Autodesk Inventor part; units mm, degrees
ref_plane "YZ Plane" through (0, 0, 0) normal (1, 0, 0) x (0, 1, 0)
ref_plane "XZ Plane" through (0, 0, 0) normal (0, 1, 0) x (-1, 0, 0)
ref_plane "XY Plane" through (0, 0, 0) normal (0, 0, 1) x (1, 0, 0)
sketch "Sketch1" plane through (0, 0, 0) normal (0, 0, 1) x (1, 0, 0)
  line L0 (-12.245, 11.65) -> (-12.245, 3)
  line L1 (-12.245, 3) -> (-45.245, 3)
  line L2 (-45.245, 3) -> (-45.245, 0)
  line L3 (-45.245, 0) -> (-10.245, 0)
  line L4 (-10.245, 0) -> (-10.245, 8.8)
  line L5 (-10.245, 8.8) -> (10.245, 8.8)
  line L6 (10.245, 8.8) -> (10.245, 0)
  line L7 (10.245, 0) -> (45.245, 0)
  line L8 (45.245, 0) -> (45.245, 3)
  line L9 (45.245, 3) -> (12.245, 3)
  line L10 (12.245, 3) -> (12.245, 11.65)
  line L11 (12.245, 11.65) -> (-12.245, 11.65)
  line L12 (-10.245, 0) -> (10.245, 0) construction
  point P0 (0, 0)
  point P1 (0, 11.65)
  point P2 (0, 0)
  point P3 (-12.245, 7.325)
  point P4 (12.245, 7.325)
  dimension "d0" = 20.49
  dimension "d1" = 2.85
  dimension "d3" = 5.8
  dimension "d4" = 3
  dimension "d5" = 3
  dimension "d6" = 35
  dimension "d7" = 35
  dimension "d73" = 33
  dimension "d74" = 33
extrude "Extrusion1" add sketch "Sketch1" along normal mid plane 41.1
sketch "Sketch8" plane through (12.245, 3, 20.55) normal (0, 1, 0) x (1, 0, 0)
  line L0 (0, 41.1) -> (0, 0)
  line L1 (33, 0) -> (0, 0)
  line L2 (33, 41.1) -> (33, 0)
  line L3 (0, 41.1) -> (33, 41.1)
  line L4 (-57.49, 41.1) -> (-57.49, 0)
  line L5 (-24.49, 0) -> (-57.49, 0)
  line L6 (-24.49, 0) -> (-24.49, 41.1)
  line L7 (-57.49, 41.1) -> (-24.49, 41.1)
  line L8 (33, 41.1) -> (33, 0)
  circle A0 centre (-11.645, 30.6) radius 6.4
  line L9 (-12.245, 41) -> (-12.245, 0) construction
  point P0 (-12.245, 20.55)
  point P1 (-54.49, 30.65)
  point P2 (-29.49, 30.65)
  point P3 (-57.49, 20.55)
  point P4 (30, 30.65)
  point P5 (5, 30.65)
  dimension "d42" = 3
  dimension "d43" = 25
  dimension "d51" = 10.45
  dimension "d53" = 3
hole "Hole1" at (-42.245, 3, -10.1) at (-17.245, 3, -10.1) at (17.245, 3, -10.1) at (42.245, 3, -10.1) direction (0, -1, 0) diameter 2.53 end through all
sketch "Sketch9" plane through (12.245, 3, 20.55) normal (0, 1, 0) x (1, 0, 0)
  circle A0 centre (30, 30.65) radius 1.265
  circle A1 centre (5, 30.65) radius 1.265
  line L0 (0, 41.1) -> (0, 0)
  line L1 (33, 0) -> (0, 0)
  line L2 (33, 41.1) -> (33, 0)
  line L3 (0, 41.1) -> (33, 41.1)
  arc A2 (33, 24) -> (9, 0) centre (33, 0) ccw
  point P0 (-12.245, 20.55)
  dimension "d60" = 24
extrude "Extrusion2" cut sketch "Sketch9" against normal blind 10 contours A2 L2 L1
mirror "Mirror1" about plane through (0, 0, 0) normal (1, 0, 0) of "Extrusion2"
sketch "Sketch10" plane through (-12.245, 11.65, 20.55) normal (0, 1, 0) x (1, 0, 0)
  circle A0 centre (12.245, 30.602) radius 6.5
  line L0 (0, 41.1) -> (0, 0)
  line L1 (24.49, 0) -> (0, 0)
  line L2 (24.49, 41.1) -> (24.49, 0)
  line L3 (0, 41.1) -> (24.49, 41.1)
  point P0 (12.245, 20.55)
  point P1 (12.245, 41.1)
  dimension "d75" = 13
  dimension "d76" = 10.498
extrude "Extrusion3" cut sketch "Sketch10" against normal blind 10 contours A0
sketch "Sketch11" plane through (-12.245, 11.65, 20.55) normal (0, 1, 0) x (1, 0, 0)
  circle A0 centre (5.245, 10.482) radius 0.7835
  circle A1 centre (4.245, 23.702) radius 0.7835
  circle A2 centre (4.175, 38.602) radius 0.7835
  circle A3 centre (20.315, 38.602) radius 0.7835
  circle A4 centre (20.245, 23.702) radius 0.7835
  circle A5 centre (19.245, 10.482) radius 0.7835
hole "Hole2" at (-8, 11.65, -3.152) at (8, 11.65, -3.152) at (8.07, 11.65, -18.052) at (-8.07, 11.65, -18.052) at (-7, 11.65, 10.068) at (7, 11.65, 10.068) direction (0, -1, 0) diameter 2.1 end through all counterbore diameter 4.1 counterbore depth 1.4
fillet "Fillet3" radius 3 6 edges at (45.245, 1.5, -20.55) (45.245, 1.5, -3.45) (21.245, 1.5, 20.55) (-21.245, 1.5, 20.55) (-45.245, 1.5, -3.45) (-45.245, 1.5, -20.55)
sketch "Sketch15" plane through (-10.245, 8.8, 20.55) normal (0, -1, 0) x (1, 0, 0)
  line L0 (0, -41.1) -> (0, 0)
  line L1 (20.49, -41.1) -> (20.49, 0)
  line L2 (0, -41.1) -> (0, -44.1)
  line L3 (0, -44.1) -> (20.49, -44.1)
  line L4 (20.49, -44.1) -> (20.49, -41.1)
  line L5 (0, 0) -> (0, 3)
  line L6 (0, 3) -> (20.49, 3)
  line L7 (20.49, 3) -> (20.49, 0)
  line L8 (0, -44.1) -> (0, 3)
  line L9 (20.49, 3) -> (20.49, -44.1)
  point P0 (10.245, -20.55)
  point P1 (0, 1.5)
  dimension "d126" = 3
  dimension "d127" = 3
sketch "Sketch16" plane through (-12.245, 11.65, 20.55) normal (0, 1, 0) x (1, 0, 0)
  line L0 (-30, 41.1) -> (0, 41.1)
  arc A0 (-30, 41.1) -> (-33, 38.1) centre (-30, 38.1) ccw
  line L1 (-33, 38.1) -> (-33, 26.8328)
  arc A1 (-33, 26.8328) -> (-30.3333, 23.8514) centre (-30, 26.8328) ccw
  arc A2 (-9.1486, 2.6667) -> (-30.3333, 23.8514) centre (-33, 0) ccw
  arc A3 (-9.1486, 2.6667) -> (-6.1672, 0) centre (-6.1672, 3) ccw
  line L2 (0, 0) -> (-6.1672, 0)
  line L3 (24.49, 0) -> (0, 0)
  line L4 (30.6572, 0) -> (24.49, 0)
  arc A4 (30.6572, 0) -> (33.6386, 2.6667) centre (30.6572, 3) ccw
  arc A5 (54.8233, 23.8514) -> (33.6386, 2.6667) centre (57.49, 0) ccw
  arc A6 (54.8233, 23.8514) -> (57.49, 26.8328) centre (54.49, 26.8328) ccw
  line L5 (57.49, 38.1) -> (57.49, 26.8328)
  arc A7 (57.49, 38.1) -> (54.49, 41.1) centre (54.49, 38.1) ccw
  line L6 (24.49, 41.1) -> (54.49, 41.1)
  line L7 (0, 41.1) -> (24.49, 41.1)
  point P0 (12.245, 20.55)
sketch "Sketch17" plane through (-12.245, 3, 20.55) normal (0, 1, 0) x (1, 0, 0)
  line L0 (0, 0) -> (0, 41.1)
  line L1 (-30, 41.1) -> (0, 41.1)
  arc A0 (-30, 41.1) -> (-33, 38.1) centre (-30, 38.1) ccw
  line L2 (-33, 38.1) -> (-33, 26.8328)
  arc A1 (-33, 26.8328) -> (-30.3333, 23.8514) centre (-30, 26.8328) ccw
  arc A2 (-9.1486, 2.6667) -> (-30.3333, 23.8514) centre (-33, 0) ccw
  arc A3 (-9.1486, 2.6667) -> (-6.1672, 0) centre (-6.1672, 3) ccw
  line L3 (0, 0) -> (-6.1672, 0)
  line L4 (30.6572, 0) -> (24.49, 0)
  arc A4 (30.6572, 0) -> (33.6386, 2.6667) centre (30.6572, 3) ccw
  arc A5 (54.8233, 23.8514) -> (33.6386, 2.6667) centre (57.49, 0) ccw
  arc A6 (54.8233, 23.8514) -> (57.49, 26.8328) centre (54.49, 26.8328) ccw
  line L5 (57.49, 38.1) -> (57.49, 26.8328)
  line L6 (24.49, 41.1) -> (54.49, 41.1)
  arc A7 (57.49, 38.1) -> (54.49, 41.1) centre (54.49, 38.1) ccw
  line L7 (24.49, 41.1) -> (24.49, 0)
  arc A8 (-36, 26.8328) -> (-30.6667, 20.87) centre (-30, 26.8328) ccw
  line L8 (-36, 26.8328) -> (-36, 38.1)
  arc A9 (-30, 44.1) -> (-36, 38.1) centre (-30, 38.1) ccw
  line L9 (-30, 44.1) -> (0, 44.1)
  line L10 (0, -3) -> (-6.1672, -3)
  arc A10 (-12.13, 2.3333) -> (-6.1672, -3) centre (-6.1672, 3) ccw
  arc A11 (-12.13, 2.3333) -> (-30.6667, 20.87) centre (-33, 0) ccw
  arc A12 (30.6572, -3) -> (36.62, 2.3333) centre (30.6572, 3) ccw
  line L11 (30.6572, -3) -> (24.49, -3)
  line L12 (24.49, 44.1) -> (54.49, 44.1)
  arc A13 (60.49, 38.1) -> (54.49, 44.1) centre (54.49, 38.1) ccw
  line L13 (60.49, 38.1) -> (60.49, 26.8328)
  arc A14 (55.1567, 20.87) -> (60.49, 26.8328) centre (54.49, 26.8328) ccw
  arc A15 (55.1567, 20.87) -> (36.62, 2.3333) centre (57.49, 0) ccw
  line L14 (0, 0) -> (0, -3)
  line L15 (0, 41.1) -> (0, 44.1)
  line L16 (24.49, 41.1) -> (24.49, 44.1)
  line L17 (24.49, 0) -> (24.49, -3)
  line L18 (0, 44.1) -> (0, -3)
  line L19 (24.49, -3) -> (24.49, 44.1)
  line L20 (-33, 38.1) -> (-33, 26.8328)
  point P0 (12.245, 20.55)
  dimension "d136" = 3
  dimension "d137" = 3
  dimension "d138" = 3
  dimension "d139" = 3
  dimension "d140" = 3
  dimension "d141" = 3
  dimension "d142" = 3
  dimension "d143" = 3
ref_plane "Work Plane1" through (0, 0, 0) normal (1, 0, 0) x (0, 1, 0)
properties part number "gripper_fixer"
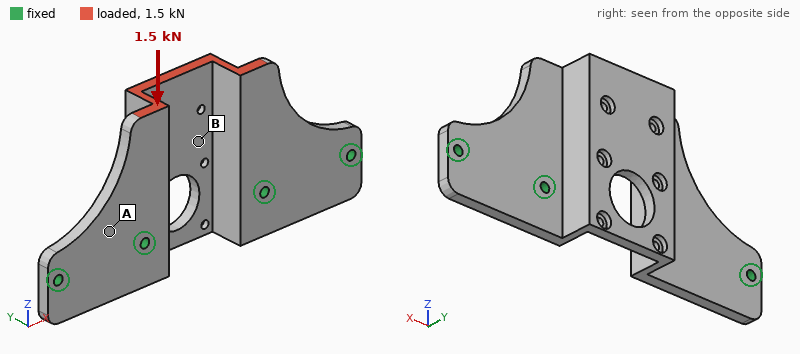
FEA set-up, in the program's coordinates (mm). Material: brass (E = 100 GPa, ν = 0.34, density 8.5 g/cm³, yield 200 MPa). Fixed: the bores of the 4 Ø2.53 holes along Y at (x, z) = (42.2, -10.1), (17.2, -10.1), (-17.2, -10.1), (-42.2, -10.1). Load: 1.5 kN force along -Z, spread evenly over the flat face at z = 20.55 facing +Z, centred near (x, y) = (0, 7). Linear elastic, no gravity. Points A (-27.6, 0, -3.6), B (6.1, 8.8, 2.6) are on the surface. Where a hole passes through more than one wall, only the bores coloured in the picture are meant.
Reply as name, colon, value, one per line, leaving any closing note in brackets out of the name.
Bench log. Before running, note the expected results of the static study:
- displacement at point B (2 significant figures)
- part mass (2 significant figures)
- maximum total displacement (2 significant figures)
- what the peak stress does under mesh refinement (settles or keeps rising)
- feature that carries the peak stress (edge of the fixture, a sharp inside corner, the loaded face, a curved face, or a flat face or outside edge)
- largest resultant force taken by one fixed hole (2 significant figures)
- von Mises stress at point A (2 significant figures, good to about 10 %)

displacement at point B: 0.050 mm
part mass: 78 g
maximum total displacement: 0.11 mm
what the peak stress does under mesh refinement: keeps rising
feature that carries the peak stress: edge of the fixture
largest resultant force taken by one fixed hole: 900 N
von Mises stress at point A: 28 MPa
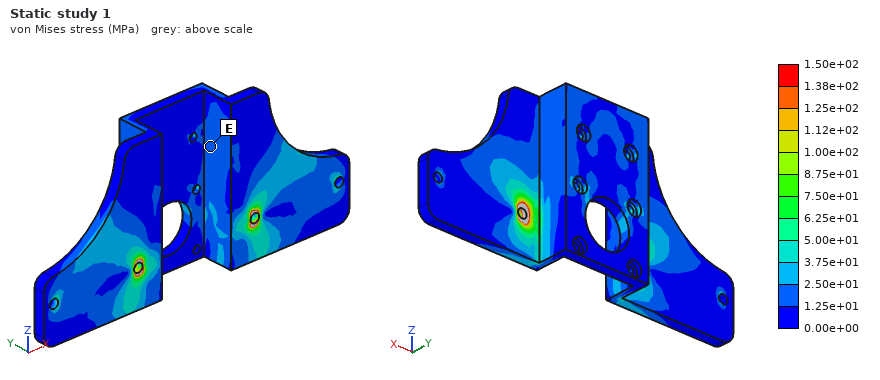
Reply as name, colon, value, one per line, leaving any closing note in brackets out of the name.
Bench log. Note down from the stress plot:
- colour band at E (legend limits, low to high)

colour band at E: 1.25e+01 to 2.50e+01 MPa
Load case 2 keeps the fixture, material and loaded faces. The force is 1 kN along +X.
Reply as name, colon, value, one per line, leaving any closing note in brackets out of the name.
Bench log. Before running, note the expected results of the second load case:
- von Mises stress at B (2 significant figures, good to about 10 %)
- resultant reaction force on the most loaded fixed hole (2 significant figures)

von Mises stress at B: 30 MPa
resultant reaction force on the most loaded fixed hole: 400 N
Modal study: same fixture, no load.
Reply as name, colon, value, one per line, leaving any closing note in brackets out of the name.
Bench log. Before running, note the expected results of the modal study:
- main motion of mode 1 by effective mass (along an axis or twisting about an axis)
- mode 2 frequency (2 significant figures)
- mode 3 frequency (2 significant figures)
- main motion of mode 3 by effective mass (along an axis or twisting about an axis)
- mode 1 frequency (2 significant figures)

main motion of mode 1 by effective mass: along Y
mode 2 frequency: 4600 Hz
mode 3 frequency: 6500 Hz
main motion of mode 3 by effective mass: along X
mode 1 frequency: 2000 Hz
